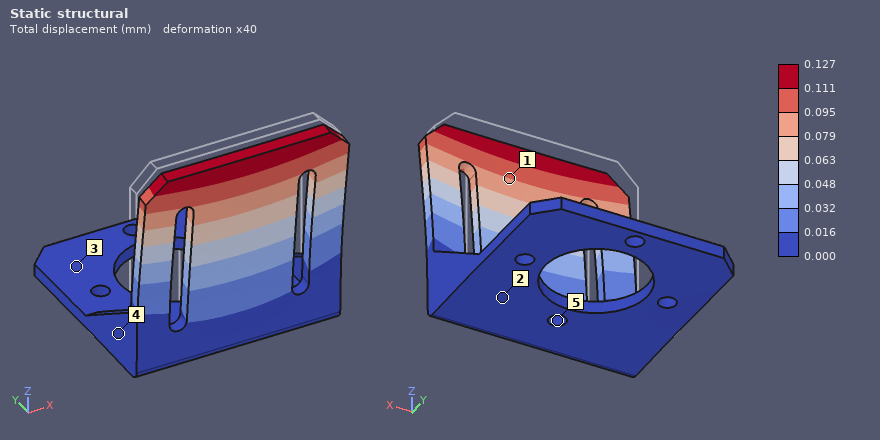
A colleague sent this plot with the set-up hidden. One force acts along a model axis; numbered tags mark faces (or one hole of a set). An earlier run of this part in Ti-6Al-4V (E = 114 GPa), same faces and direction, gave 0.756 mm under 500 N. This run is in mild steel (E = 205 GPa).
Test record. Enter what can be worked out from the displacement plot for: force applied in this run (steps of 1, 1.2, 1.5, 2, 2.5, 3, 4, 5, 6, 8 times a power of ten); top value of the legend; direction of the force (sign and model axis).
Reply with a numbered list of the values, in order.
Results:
1. 150 N
2. 0.127 mm
3. -Y
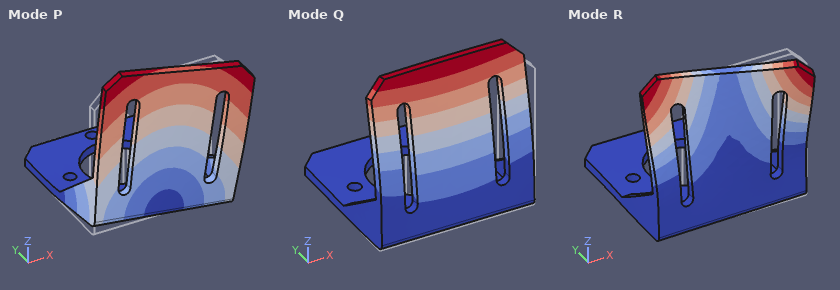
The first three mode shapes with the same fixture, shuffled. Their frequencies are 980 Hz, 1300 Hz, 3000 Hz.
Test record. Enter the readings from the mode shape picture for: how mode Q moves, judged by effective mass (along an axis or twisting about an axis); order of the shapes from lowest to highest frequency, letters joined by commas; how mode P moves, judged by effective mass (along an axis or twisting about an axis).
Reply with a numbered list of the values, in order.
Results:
1. along Y
2. Q, P, R
3. along X
